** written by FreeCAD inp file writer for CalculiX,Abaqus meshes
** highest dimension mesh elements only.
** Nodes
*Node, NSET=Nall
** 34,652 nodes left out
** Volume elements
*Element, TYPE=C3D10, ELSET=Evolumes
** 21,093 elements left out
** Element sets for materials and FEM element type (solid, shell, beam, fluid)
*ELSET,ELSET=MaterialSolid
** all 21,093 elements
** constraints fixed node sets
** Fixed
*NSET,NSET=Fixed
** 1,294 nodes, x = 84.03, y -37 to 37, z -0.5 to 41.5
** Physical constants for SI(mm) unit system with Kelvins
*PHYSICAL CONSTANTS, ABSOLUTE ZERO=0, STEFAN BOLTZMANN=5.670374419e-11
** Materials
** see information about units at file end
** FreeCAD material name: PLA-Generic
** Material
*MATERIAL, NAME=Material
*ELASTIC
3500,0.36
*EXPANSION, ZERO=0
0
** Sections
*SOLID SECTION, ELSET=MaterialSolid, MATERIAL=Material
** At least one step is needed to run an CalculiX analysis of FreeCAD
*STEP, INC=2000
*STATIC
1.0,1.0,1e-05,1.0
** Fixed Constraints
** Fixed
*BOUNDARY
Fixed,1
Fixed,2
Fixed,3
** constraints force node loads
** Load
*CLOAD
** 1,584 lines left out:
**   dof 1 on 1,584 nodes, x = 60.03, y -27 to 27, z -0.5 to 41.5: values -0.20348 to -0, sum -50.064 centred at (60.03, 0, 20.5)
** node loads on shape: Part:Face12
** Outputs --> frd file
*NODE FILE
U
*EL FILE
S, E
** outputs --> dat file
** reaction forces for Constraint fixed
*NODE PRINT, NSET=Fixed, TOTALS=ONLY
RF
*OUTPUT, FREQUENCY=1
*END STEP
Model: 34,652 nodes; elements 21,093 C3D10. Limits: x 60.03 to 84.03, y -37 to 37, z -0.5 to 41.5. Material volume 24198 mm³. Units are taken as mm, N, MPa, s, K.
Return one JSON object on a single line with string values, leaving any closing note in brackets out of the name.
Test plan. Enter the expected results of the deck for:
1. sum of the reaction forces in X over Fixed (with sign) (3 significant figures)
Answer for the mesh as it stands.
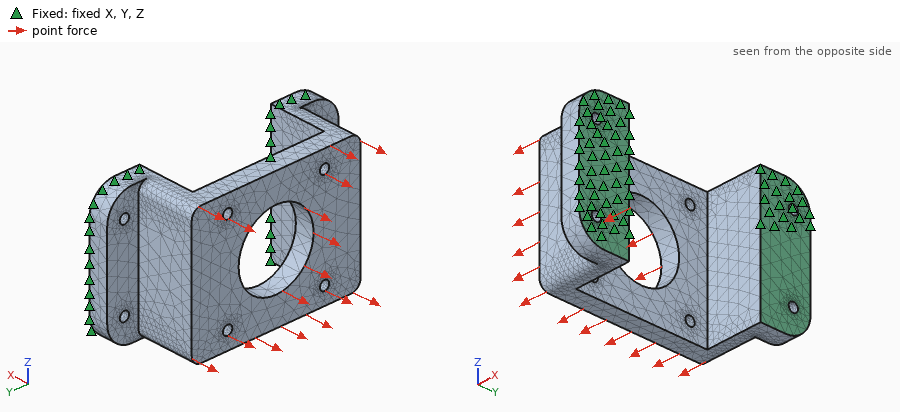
{"sum of the reaction forces in X over Fixed (with sign)": "50.1 N"}
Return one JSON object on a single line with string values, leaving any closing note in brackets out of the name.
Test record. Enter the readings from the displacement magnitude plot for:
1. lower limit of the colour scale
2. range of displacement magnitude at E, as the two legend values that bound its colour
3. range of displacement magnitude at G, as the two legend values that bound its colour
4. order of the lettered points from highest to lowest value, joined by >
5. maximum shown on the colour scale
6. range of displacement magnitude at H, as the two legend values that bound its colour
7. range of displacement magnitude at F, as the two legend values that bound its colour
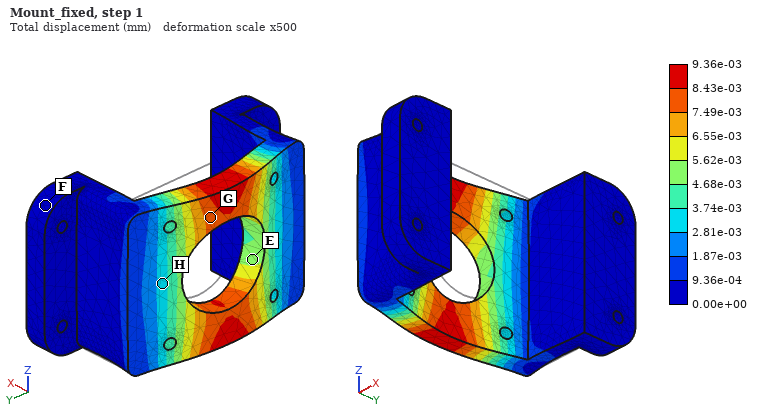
{"lower limit of the colour scale": "0.00e+00 mm", "range of displacement magnitude at E, as the two legend values that bound its colour": "4.68e-03 to 5.62e-03 mm", "range of displacement magnitude at G, as the two legend values that bound its colour": "7.49e-03 to 8.43e-03 mm", "order of the lettered points from highest to lowest value, joined by >": "G > E > H > F", "maximum shown on the colour scale": "9.36e-03 mm", "range of displacement magnitude at H, as the two legend values that bound its colour": "2.81e-03 to 3.74e-03 mm", "range of displacement magnitude at F, as the two legend values that bound its colour": "0.00e+00 to 9.36e-04 mm"}
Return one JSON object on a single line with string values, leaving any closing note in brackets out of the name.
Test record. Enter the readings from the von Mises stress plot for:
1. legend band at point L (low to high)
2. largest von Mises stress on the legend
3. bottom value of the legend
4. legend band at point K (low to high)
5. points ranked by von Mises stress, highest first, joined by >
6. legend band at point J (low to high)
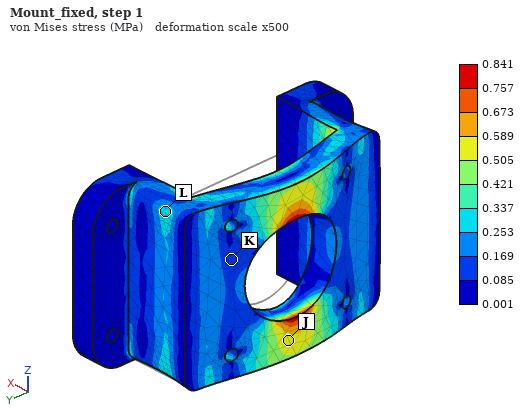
{"legend band at point L": "0.253 to 0.337 MPa", "largest von Mises stress on the legend": "0.841 MPa", "bottom value of the legend": "0.001 MPa", "legend band at point K": "0.085 to 0.169 MPa", "points ranked by von Mises stress, highest first, joined by >": "J > L > K", "legend band at point J": "0.505 to 0.589 MPa"}
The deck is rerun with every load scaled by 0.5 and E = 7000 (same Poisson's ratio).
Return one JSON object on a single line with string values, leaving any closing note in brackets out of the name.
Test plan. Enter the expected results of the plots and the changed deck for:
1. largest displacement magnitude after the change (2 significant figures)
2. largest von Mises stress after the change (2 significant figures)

{"largest displacement magnitude after the change": "0.0023 mm", "largest von Mises stress after the change": "0.42 MPa"}
